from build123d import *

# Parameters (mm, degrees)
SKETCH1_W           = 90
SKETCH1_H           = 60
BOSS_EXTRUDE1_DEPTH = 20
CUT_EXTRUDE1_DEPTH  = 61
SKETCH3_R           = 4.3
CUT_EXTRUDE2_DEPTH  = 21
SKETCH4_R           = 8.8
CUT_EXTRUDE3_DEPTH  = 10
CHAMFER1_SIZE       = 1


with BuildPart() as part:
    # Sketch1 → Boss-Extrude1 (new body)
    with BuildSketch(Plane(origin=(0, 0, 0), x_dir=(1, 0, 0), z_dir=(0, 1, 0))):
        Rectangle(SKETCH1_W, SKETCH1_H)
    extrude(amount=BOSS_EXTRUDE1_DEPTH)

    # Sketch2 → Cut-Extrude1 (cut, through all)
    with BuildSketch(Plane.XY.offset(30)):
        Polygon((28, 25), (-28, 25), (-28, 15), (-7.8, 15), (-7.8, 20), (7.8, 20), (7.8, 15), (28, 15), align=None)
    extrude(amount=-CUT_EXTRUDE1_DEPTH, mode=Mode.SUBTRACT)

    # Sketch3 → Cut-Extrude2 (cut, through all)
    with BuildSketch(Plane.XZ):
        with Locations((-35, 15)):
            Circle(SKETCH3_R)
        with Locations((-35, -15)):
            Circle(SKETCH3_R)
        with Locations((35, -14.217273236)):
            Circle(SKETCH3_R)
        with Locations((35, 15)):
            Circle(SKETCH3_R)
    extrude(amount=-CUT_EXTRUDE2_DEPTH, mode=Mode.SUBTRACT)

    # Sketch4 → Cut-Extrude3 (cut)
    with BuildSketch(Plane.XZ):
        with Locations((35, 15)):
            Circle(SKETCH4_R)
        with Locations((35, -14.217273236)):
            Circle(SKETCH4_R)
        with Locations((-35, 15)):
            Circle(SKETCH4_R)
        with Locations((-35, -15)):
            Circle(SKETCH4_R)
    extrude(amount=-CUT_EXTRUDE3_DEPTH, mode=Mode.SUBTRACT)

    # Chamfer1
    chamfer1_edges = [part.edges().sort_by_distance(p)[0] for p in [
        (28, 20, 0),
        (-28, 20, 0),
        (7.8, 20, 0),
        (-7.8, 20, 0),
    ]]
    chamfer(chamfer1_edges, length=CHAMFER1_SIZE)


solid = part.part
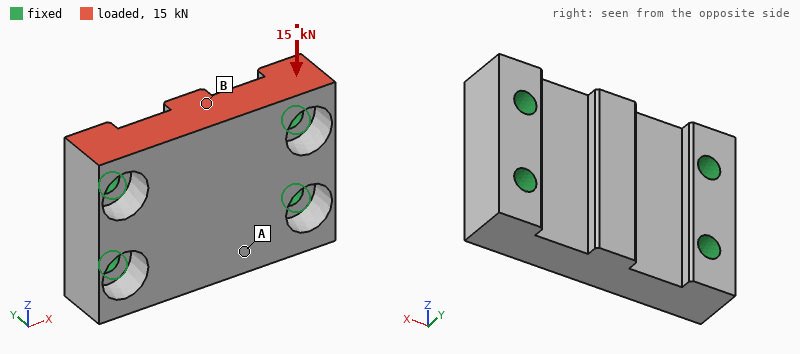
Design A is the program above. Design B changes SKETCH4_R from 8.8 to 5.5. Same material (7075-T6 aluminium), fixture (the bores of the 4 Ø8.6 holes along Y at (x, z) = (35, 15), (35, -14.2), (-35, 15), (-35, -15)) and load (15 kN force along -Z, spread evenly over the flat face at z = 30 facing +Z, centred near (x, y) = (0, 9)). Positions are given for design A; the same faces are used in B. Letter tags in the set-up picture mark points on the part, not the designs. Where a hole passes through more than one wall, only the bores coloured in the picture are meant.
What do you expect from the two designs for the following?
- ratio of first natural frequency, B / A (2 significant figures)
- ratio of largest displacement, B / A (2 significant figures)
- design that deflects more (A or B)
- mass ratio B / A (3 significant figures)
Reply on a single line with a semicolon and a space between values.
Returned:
1.0; 0.66; A; 1.07
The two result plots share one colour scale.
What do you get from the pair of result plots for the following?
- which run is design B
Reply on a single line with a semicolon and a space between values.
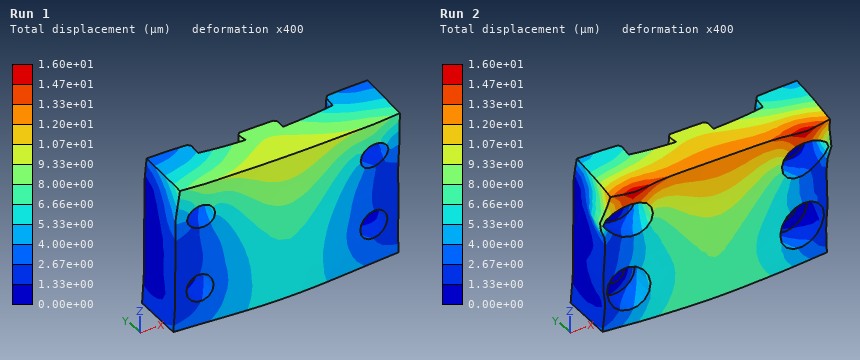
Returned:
Run 1
